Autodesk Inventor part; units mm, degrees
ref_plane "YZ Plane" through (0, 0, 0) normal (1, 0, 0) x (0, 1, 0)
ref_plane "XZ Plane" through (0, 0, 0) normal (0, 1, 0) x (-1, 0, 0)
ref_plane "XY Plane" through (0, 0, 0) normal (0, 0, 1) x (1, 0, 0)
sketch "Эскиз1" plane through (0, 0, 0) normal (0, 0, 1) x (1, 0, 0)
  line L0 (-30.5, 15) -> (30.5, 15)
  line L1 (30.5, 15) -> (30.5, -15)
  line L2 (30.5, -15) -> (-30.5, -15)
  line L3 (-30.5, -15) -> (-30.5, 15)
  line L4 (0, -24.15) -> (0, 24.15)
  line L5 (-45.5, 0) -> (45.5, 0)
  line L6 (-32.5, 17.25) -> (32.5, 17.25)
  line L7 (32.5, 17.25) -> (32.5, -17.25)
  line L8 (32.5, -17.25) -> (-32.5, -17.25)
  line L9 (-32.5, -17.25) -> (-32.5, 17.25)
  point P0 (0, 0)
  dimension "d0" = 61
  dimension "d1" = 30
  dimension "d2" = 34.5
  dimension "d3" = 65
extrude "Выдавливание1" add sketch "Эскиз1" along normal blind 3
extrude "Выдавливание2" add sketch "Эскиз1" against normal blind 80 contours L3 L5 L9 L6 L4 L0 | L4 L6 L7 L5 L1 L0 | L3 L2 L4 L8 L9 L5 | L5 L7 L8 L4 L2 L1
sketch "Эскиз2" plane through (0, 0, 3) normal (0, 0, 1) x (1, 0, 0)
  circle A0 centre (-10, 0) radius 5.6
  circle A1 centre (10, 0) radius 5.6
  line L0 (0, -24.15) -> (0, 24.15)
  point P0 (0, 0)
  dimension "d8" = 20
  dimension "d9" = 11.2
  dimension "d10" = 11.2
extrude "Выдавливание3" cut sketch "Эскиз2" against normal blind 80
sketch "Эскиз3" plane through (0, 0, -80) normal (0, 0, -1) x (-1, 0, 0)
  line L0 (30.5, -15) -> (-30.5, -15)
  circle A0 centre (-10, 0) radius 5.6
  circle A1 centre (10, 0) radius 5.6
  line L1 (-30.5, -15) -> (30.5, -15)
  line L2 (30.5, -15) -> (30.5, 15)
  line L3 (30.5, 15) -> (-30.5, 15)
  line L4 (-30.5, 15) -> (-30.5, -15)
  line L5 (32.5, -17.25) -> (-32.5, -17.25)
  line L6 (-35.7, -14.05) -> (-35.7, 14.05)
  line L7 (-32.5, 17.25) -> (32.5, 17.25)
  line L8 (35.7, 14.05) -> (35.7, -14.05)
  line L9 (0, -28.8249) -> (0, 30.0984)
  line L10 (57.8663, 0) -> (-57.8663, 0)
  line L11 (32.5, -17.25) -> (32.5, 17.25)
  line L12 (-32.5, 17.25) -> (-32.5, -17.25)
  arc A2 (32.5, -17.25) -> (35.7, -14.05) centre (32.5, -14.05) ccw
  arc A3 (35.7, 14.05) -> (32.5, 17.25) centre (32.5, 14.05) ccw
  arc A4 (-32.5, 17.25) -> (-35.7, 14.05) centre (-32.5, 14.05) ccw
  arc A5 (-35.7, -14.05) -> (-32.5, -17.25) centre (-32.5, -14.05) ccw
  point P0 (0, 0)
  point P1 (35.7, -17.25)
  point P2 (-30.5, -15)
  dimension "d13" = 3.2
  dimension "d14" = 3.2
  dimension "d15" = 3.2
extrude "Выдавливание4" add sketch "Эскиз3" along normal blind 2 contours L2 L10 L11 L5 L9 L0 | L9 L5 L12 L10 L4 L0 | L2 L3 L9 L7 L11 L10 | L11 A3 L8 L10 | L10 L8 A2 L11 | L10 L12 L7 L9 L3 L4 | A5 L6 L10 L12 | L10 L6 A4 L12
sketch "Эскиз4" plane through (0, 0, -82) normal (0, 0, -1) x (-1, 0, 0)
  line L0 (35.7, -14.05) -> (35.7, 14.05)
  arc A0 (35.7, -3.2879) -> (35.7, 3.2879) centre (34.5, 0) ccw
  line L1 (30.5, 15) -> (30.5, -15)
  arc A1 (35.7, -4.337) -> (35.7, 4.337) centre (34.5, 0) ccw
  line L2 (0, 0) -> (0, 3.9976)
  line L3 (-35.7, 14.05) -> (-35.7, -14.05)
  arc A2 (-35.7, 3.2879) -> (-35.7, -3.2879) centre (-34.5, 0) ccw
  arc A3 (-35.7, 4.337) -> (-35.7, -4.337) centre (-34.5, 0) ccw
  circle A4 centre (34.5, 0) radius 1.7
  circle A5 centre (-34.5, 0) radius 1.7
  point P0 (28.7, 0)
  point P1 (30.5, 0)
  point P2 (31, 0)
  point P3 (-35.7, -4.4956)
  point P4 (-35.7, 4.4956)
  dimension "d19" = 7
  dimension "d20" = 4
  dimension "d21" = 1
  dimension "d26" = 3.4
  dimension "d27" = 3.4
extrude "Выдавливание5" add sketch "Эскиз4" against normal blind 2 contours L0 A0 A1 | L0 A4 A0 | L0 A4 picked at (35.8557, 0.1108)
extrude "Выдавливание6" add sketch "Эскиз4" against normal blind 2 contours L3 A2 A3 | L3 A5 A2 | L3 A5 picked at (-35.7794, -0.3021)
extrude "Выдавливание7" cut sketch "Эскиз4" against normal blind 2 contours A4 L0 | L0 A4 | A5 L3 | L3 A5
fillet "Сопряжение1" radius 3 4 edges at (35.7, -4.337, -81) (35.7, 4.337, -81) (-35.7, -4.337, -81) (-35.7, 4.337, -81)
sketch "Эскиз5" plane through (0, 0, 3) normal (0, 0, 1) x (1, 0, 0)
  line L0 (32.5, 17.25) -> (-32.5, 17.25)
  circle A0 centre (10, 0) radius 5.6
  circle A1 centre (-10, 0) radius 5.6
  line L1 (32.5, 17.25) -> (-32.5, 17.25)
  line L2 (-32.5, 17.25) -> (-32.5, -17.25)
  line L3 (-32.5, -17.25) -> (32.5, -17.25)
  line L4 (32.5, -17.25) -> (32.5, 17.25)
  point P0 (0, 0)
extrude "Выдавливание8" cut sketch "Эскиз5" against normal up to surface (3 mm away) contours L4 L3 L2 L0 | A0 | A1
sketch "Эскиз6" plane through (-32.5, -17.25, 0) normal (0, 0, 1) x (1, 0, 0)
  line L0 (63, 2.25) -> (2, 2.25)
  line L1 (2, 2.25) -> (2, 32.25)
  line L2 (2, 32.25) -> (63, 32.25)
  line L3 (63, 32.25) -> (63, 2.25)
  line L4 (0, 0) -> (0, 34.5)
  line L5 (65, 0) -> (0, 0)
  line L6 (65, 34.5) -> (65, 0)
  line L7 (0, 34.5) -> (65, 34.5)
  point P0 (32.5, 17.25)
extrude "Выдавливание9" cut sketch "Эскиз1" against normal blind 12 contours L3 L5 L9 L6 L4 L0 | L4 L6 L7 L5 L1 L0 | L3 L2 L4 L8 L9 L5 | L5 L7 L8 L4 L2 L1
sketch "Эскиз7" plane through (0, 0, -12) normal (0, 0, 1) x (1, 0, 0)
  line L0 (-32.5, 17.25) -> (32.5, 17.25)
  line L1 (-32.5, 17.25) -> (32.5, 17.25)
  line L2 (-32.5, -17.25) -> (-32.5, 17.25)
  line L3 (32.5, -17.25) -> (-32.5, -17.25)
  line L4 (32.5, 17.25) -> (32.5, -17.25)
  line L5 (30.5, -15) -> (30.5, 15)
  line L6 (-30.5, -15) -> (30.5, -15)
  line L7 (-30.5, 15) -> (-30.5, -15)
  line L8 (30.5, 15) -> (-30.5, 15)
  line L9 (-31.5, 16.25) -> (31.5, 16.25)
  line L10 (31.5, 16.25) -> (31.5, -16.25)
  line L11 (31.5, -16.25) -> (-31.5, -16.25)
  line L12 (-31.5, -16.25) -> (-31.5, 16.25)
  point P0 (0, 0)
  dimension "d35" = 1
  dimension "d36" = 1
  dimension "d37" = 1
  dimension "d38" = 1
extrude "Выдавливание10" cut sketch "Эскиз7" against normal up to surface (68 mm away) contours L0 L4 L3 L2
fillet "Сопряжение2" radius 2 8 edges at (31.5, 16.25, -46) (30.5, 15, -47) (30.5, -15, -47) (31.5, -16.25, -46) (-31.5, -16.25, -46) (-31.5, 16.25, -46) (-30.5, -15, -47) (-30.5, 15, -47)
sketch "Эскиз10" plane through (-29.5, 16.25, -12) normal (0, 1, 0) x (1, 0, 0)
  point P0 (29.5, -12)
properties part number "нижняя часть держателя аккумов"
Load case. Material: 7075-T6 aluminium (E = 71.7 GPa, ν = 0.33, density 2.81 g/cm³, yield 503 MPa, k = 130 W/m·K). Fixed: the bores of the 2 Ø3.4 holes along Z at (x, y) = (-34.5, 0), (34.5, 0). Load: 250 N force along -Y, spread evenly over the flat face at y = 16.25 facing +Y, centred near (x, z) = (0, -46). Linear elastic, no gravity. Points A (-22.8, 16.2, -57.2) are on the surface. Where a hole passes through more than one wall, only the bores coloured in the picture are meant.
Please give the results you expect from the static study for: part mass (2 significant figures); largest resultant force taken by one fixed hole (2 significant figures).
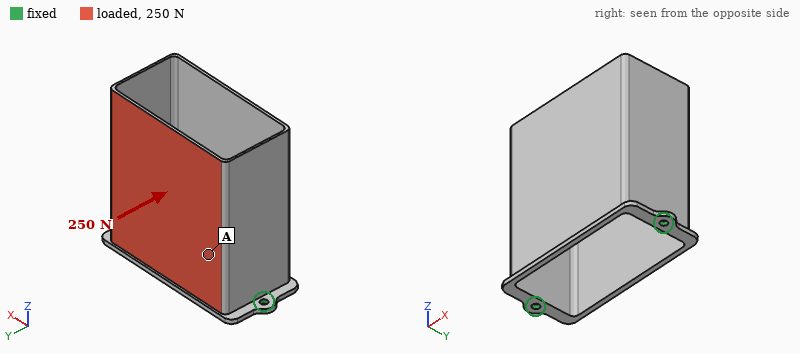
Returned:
45 g
130 N
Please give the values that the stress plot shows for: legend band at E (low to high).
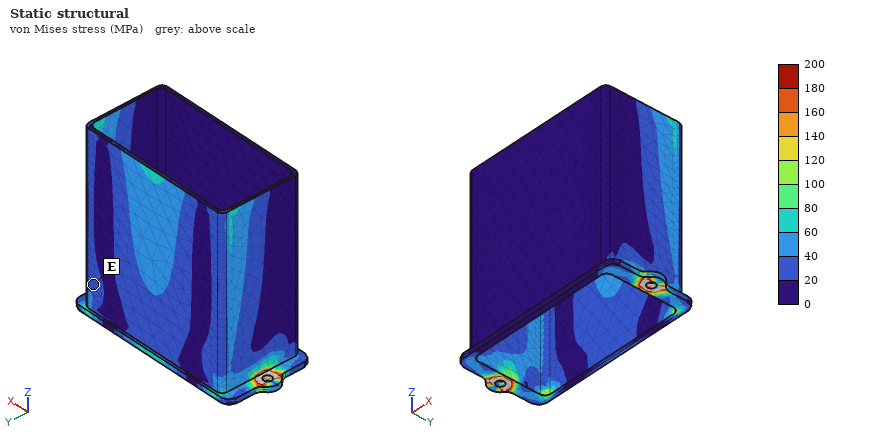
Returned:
20 to 40 MPa
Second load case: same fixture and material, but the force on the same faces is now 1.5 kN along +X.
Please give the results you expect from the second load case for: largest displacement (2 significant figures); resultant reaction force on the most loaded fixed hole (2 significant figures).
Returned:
0.80 mm
1.1 kN
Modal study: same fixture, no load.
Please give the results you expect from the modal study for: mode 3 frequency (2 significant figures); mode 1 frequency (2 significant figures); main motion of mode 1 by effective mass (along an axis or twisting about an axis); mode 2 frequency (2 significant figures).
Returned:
1100 Hz
500 Hz
along Y
1000 Hz
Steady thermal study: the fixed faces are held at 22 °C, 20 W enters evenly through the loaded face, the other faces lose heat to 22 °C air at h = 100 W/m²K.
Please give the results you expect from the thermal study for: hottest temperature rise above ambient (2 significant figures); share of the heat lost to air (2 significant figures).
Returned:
22 K
83 %
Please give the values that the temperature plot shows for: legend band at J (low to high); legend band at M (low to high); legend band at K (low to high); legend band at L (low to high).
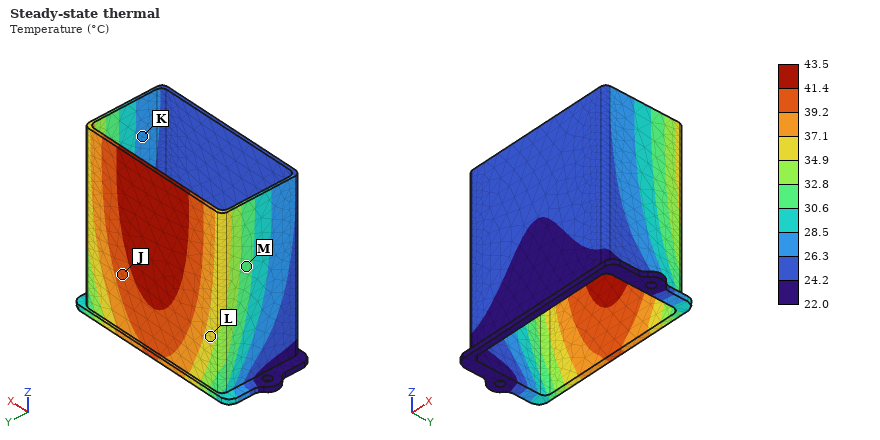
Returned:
39.2 to 41.4 °C
30.6 to 32.8 °C
26.3 to 28.5 °C
34.9 to 37.1 °C
